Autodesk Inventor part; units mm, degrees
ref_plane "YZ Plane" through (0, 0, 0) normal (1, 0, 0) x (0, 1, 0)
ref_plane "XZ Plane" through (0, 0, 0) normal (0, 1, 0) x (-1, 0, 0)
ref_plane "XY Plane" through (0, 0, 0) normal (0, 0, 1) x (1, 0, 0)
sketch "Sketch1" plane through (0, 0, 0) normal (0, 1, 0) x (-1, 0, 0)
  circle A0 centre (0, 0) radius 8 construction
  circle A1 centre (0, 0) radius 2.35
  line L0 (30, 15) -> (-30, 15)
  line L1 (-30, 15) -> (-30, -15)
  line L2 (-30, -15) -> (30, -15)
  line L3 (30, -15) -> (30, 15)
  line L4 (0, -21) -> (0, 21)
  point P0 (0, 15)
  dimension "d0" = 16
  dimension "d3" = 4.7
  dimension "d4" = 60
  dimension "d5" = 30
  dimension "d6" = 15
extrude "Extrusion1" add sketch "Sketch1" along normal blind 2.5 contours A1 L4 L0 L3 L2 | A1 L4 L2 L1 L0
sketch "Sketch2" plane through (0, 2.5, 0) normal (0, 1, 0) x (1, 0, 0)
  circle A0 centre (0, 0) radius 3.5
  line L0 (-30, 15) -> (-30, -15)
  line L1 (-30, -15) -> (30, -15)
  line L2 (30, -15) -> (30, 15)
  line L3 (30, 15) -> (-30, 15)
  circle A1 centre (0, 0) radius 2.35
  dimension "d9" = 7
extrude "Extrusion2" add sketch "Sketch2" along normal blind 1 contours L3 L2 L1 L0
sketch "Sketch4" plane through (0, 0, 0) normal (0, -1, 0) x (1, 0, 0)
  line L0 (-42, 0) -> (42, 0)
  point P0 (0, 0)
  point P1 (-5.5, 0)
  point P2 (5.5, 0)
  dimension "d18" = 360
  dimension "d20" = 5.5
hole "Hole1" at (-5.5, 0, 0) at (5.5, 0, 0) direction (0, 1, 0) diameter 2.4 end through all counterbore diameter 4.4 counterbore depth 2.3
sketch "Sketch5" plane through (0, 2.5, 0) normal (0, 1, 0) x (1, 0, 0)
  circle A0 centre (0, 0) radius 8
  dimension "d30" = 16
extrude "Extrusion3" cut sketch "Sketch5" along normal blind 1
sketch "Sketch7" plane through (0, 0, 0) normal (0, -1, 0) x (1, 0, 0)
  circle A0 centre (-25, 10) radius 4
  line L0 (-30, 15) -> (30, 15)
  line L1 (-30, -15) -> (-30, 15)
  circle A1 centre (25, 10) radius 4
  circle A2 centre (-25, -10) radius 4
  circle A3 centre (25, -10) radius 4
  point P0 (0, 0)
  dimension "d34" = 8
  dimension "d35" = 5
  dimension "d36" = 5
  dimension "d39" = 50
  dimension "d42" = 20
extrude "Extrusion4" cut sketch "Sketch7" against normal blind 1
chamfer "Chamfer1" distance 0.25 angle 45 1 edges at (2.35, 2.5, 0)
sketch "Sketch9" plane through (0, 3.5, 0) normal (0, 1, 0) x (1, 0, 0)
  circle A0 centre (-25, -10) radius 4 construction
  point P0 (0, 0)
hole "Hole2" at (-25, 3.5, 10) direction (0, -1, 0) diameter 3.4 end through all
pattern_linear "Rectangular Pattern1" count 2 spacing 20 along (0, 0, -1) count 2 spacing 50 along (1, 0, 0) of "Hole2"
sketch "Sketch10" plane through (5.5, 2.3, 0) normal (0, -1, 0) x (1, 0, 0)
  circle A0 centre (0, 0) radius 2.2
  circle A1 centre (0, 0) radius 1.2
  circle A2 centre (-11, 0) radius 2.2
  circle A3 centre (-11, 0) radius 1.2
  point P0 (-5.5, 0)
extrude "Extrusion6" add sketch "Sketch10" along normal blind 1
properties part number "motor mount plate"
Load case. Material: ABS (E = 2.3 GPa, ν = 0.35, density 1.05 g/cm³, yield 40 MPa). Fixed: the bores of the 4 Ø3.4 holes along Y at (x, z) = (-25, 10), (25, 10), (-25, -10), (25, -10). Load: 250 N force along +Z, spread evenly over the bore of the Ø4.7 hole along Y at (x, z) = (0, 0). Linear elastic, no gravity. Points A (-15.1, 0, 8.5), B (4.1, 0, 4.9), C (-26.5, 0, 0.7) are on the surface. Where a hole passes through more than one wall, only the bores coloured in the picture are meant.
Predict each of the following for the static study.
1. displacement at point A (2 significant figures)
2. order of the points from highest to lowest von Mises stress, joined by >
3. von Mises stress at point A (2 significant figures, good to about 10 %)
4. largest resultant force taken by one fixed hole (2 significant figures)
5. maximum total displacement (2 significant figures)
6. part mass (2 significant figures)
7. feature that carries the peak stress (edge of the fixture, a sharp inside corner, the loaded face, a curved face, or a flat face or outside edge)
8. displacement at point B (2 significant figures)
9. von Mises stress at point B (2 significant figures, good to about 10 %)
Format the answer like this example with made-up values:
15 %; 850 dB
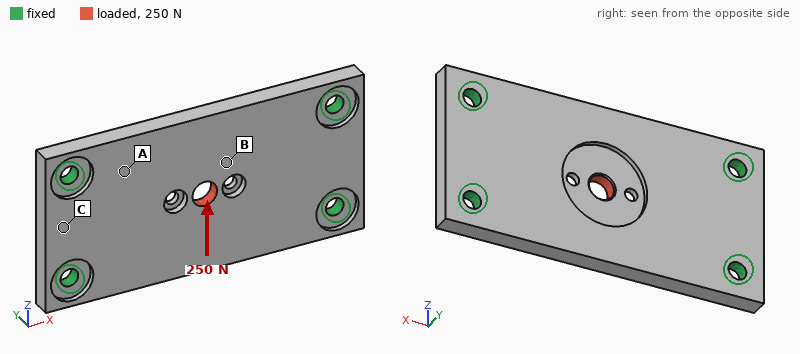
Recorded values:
25 µm; B > A > C; 2.7 MPa; 91 N; 70 µm; 6.0 g; the loaded face; 55 µm; 4.4 MPa
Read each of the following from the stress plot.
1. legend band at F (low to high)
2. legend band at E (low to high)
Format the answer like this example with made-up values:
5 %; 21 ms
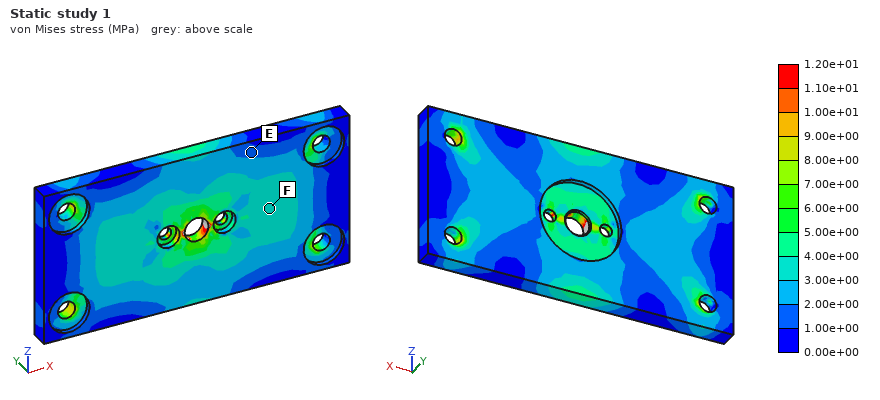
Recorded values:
3.00e+00 to 4.00e+00 MPa; 1.00e+00 to 2.00e+00 MPa
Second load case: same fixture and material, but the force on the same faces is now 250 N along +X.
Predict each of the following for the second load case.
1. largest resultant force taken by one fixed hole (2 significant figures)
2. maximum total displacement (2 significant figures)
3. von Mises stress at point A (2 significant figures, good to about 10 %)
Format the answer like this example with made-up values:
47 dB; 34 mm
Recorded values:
64 N; 51 µm; 1.5 MPa
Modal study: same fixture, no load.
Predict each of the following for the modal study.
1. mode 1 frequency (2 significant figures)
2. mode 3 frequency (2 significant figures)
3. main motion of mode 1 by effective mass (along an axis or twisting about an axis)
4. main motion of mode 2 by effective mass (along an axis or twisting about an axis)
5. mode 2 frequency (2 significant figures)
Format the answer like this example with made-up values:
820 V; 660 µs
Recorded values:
1800 Hz; 4800 Hz; along Y; twisting about X; 2800 Hz
